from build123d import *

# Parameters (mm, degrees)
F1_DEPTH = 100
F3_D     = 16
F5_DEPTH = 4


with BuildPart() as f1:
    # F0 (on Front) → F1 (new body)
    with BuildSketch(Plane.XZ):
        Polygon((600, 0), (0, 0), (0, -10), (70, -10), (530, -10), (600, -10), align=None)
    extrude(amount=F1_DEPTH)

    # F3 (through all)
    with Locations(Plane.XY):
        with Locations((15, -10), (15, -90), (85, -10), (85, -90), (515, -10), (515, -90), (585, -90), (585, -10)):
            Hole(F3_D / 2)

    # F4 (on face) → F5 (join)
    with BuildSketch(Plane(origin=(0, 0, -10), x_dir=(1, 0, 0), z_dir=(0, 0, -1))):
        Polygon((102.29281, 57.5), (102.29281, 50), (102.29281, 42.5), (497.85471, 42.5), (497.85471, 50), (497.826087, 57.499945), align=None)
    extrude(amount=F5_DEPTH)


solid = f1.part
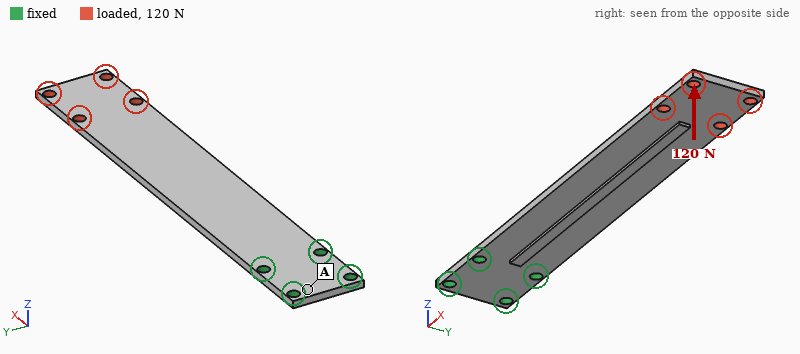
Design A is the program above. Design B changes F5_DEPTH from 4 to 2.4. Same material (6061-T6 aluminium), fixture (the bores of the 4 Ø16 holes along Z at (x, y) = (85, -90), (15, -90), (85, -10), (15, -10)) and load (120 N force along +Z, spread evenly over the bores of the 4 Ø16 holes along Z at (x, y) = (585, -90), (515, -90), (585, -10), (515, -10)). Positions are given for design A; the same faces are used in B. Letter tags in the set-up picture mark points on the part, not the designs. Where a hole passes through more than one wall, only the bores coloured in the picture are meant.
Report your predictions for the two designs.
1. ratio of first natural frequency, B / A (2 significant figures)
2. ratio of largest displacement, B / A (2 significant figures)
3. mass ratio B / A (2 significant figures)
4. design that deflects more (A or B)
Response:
0.95
1.1
0.98
B
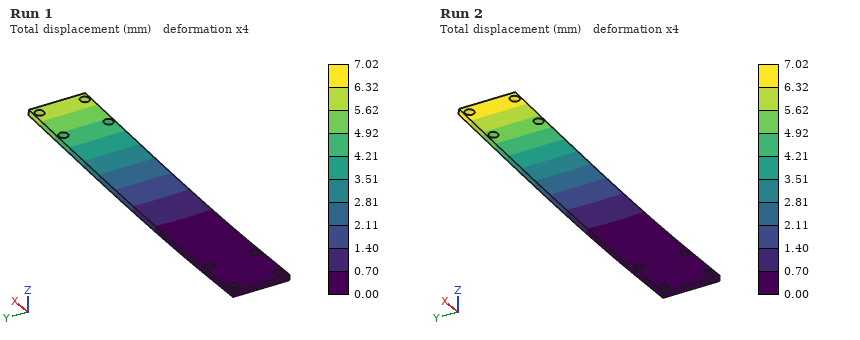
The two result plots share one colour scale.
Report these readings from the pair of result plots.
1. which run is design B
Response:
Run 2
